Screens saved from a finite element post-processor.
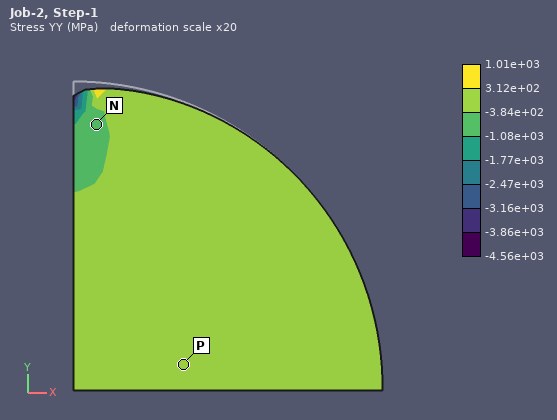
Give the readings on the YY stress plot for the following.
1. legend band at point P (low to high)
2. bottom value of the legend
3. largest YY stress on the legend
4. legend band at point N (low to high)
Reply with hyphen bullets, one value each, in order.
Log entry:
- -3.84e+02 to 3.12e+02 MPa
- -4.56e+03 MPa
- 1.01e+03 MPa
- -1.08e+03 to -3.84e+02 MPa
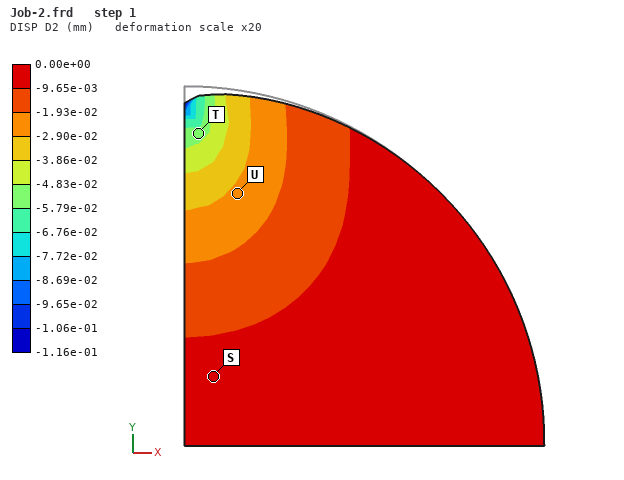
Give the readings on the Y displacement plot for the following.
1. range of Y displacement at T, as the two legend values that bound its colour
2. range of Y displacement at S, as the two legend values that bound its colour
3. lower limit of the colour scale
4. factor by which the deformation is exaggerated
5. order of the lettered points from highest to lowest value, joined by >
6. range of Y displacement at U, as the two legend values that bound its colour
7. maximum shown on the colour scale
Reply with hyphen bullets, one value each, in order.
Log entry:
- -5.79e-02 to -4.83e-02 mm
- -9.65e-03 to 0.00e+00 mm
- -1.16e-01 mm
- 20
- S > U > T
- -2.90e-02 to -1.93e-02 mm
- 0.00e+00 mm
